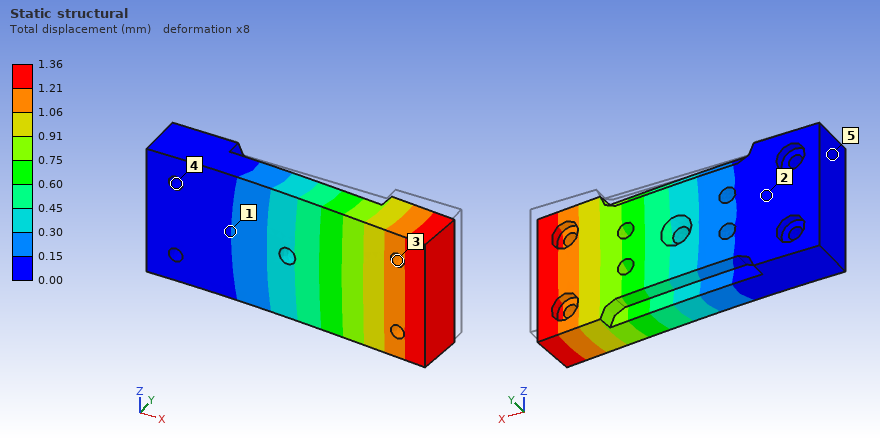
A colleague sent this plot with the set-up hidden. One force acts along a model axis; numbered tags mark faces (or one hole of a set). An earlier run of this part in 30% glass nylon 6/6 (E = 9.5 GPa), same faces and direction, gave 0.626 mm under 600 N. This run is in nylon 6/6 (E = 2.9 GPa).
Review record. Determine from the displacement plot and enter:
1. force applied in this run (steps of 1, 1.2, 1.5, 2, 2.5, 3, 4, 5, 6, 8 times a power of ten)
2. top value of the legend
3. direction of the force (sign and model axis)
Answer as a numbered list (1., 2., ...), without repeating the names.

1. 400 N
2. 1.36 mm
3. -Y
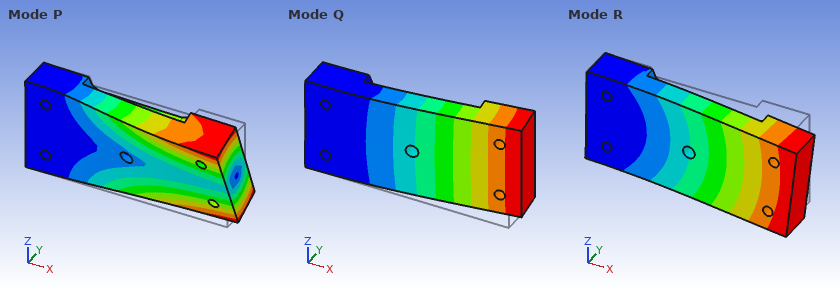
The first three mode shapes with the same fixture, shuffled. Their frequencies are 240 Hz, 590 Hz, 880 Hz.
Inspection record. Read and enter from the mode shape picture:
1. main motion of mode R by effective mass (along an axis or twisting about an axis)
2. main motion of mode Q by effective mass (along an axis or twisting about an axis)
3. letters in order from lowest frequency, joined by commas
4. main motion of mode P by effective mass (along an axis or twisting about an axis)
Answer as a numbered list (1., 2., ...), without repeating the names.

1. along Z
2. along Y
3. Q, R, P
4. twisting about X
